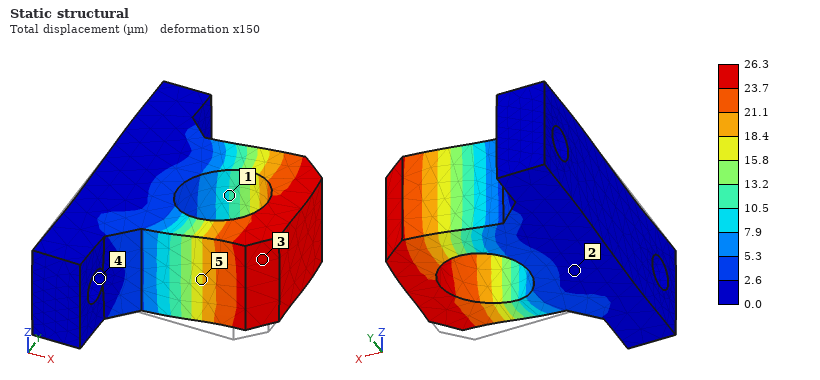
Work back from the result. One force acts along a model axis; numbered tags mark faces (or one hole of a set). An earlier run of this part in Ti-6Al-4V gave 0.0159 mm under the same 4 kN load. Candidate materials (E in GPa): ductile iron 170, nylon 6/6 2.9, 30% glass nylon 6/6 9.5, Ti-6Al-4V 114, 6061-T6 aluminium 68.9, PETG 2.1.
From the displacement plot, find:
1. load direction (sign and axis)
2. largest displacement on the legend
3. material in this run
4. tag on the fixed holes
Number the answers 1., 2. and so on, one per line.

1. +Y
2. 26.3 µm
3. 6061-T6 aluminium
4. 4
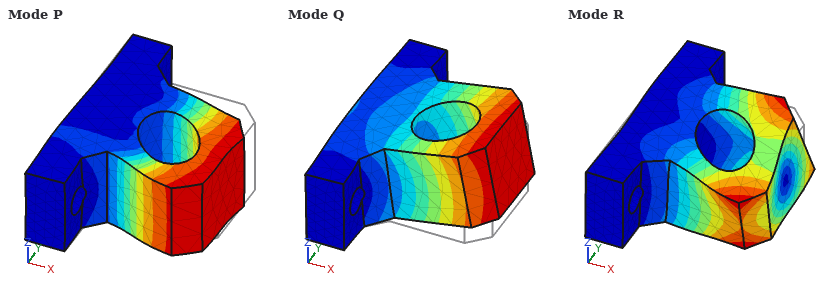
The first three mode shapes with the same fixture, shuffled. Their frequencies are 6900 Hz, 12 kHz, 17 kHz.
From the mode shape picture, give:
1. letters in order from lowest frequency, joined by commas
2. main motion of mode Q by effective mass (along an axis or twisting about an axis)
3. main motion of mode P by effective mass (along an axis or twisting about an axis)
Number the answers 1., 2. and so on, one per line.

1. Q, P, R
2. along Z
3. along Y
